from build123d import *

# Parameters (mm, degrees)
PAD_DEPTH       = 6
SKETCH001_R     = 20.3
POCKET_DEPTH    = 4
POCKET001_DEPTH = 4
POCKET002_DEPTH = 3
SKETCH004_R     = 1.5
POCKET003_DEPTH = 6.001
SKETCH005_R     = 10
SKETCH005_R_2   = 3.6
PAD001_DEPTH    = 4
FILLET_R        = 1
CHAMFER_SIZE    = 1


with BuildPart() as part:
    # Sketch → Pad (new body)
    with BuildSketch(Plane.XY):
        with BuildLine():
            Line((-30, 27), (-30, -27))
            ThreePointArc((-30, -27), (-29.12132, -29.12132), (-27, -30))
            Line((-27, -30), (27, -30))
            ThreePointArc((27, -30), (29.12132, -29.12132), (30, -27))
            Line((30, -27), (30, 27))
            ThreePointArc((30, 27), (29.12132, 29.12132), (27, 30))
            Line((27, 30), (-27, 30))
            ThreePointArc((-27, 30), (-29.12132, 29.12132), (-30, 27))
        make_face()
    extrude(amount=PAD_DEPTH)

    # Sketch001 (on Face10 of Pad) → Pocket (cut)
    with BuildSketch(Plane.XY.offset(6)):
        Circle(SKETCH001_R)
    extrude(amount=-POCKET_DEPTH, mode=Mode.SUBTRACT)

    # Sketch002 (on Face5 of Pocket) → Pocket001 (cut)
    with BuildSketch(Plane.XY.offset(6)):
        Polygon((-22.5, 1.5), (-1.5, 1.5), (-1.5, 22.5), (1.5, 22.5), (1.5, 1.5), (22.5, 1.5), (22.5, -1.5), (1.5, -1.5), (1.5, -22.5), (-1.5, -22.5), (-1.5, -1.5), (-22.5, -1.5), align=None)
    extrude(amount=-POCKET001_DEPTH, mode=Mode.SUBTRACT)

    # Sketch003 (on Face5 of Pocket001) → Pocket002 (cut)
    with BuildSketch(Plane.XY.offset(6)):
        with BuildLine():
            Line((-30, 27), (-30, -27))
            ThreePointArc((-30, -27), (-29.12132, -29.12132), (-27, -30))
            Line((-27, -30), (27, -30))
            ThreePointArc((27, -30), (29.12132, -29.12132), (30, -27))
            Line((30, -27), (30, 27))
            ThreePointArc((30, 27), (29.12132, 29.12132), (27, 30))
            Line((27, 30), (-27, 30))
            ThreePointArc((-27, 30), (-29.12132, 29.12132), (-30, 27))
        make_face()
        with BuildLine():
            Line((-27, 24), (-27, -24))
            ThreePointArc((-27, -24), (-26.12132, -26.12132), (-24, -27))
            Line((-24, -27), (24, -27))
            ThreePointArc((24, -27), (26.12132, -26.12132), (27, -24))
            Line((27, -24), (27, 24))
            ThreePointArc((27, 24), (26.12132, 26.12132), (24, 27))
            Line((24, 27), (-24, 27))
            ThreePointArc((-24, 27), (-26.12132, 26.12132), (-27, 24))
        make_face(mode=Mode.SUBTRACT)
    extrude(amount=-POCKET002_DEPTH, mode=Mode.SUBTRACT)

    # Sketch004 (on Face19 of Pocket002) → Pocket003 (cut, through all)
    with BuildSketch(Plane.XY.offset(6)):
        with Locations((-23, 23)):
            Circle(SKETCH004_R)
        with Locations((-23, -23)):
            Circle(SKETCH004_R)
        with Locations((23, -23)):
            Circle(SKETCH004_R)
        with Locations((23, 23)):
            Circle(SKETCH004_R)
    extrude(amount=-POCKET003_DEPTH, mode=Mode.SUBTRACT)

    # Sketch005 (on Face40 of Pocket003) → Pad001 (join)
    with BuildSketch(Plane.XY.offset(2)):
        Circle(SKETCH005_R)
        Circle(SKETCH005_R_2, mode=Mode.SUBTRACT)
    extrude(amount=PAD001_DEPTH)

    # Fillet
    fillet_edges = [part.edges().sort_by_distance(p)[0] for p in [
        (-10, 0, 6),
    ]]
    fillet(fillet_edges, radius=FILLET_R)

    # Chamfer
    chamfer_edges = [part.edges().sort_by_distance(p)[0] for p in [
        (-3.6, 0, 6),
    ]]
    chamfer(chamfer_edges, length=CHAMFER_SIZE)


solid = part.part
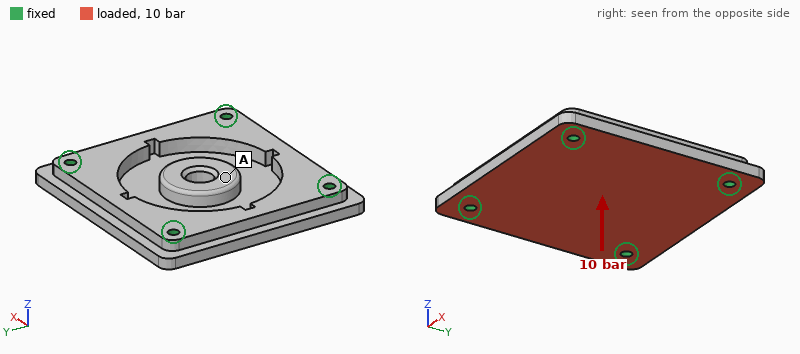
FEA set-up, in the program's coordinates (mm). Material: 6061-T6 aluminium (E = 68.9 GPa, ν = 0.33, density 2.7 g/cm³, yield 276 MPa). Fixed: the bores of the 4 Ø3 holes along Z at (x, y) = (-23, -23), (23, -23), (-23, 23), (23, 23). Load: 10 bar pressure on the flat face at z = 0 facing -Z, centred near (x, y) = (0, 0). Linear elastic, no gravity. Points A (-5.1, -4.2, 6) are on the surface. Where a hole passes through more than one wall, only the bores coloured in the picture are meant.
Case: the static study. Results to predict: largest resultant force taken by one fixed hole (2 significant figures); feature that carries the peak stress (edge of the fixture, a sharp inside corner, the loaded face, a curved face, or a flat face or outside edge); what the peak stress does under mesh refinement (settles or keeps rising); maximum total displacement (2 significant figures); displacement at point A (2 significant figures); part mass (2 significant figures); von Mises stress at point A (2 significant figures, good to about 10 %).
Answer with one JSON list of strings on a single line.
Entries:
["1.0 kN", "edge of the fixture", "keeps rising", "62 µm", "60 µm", "41 g", "12 MPa"]
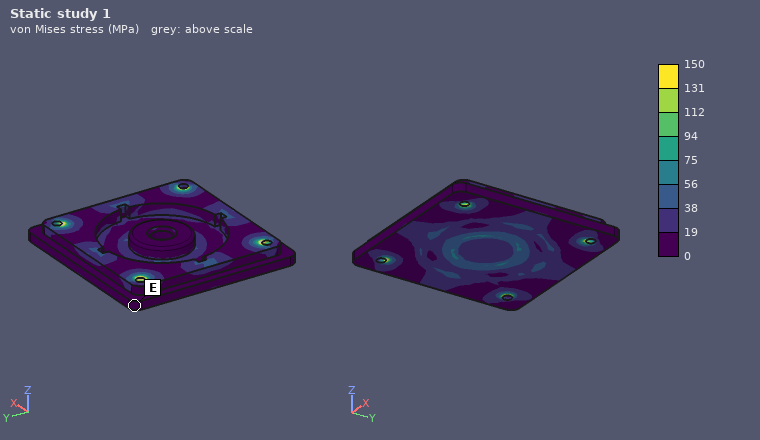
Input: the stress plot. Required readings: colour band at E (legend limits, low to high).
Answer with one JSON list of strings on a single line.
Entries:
["0 to 19 MPa"]
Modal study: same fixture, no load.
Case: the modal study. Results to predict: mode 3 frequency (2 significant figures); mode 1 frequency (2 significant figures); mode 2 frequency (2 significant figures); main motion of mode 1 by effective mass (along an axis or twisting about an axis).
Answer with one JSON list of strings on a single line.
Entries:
["12 kHz", "7800 Hz", "12 kHz", "along Z"]
